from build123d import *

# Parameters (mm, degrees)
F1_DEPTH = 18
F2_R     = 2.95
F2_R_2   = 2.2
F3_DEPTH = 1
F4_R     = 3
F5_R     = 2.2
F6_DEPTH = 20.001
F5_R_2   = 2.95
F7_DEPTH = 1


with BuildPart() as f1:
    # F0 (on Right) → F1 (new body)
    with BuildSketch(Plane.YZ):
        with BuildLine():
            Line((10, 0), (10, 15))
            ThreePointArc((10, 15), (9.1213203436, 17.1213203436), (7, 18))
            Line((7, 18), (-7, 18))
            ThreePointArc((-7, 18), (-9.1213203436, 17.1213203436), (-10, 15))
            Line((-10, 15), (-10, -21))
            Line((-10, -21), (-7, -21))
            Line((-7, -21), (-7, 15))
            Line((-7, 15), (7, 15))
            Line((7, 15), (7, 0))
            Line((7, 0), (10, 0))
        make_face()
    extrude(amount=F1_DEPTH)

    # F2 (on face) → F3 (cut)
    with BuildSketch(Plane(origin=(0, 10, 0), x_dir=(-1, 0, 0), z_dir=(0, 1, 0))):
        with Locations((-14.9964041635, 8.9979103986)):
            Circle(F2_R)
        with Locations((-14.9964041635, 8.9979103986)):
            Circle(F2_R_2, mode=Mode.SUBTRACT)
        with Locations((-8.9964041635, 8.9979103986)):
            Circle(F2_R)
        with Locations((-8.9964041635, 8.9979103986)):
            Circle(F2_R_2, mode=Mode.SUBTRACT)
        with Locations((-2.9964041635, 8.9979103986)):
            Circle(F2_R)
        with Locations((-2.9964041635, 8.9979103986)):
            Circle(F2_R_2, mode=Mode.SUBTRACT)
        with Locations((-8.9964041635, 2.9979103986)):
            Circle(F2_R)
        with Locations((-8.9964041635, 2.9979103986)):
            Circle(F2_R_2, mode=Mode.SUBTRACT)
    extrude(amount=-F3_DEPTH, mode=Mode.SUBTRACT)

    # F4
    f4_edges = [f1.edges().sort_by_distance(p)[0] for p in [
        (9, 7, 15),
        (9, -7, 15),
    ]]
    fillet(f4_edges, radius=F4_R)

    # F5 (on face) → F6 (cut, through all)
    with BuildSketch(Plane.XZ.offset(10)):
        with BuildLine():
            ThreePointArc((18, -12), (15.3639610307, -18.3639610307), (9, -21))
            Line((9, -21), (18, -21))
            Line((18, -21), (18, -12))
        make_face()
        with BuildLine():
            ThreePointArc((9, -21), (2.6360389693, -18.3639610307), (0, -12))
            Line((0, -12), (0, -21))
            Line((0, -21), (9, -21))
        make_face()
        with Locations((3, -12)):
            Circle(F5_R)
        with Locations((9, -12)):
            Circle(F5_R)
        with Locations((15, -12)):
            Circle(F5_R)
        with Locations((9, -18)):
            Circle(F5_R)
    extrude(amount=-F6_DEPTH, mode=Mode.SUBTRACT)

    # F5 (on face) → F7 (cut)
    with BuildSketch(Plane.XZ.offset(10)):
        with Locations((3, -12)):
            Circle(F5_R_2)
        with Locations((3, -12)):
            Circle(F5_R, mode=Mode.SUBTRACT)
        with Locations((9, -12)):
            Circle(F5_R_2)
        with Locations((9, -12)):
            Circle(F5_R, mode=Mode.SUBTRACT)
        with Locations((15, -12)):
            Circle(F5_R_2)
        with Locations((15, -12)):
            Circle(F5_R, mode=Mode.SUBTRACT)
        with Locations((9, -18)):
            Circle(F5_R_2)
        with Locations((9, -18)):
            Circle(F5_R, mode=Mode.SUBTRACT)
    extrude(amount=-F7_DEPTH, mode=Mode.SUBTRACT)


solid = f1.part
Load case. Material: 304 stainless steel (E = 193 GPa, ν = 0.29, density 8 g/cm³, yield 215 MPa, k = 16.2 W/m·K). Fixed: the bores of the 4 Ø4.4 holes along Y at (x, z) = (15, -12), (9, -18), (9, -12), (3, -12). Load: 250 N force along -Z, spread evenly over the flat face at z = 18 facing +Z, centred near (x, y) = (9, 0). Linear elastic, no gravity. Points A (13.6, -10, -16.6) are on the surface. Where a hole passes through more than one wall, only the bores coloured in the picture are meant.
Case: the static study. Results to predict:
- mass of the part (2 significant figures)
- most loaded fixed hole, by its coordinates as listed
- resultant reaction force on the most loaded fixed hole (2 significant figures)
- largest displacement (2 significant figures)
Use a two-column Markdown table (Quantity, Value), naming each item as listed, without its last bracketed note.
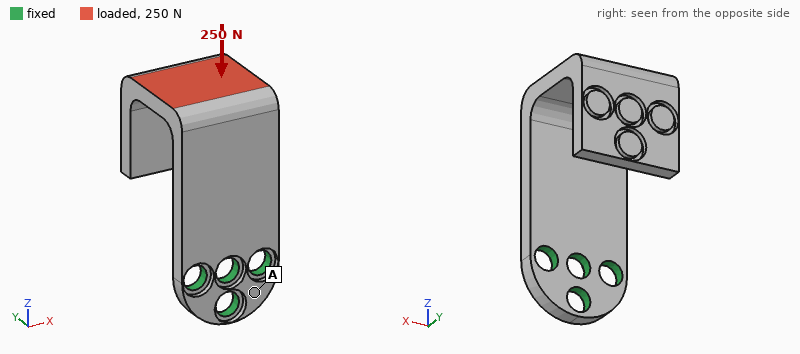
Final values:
| Quantity | Value |
|---|---|
| mass of the part | 28 g |
| most loaded fixed hole, by its coordinates as listed | (9, -12) |
| resultant reaction force on the most loaded fixed hole | 110 N |
| largest displacement | 0.18 mm |
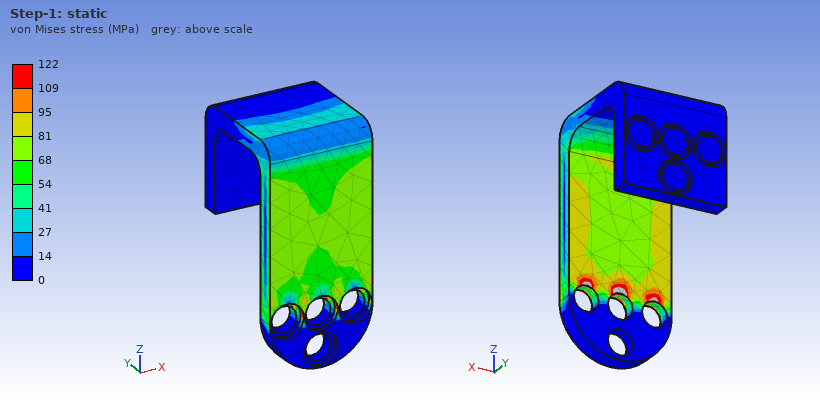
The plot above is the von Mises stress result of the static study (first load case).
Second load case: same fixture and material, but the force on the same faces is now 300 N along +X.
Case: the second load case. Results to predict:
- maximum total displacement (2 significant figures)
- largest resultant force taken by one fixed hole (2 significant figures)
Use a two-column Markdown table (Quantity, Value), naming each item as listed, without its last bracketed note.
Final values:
| Quantity | Value |
|---|---|
| maximum total displacement | 0.11 mm |
| largest resultant force taken by one fixed hole | 650 N |
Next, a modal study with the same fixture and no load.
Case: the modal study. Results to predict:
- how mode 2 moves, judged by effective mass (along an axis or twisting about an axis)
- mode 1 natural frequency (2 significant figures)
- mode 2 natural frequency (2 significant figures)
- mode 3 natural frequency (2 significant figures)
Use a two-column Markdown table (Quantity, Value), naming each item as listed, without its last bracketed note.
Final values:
| Quantity | Value |
|---|---|
| how mode 2 moves, judged by effective mass | along X |
| mode 1 natural frequency | 1100 Hz |
| mode 2 natural frequency | 1900 Hz |
| mode 3 natural frequency | 2600 Hz |
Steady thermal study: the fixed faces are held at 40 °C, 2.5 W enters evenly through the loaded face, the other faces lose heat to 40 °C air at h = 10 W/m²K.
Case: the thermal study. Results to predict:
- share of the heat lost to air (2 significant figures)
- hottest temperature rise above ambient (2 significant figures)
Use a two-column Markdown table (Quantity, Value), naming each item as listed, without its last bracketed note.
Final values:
| Quantity | Value |
|---|---|
| share of the heat lost to air | 39 % |
| hottest temperature rise above ambient | 60 K |
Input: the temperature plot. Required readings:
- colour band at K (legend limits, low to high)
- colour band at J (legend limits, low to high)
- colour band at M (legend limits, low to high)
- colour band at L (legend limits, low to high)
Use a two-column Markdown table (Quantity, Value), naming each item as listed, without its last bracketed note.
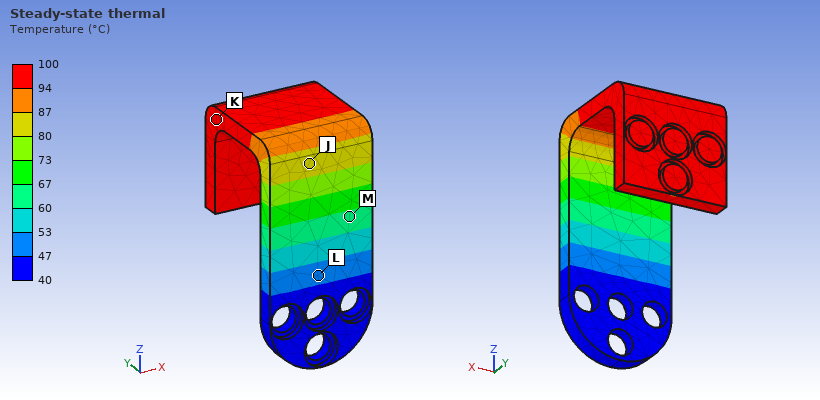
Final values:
| Quantity | Value |
|---|---|
| colour band at K | 94 to 100 °C |
| colour band at J | 80 to 87 °C |
| colour band at M | 60 to 67 °C |
| colour band at L | 47 to 53 °C |
